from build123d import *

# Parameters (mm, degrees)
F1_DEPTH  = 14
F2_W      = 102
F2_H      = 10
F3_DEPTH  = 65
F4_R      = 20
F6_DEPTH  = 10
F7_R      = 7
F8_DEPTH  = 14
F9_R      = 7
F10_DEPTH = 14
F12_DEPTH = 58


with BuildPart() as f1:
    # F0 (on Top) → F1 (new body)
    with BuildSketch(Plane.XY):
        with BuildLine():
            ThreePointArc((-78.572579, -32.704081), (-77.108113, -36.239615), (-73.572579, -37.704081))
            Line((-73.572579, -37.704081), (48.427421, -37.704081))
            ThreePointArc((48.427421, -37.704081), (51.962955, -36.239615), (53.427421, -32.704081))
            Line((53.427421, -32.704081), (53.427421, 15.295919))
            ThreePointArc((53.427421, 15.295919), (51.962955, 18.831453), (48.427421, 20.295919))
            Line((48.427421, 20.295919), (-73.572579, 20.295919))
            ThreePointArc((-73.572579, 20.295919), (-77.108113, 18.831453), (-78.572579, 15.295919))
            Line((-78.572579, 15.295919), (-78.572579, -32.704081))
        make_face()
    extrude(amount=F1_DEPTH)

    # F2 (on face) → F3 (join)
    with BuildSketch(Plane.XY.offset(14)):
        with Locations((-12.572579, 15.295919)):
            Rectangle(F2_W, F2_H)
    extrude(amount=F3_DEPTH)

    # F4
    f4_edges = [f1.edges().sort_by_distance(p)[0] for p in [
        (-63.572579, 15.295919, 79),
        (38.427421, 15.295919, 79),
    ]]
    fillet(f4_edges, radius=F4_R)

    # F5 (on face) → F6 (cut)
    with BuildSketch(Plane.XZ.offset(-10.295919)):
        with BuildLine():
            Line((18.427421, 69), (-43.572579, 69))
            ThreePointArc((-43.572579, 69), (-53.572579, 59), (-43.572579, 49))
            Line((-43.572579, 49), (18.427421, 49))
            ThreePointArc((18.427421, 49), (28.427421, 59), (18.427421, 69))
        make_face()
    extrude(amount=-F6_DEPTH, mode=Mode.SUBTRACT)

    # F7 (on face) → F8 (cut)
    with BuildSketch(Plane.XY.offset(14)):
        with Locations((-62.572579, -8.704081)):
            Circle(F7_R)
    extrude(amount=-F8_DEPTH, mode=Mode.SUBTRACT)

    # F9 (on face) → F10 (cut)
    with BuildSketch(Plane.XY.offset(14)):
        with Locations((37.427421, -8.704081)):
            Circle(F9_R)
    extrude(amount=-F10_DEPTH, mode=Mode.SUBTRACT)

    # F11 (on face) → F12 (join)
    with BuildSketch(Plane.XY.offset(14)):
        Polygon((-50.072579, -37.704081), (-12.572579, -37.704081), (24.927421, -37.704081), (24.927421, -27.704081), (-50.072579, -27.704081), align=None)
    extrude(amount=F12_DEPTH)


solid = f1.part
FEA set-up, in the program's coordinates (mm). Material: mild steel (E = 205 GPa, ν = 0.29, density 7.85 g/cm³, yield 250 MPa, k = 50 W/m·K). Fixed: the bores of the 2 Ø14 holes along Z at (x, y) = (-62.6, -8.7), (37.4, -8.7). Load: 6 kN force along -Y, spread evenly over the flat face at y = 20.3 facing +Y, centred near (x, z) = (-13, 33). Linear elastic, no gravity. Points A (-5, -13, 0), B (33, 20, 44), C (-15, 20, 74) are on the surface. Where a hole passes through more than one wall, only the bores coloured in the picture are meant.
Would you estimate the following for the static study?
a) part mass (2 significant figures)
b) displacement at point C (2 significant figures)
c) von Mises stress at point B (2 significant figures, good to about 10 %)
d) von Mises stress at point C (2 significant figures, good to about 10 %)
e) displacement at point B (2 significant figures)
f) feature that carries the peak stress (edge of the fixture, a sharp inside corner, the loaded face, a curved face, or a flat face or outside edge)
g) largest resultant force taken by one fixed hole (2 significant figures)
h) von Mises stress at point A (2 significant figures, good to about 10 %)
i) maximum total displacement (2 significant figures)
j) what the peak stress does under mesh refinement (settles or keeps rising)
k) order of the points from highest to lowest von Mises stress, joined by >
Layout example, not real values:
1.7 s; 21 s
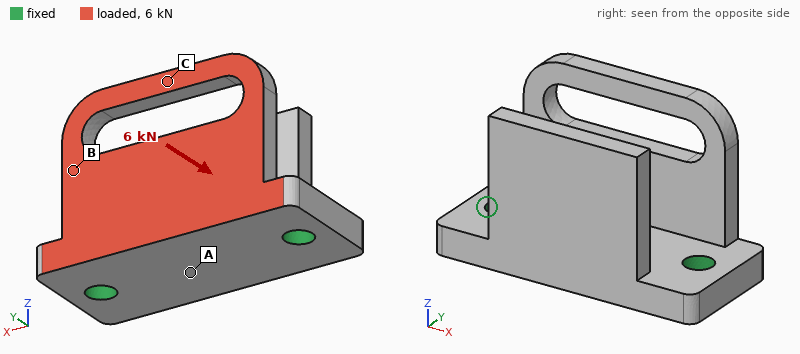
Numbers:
1.5 kg; 0.18 mm; 51 MPa; 30 MPa; 0.063 mm; a sharp inside corner; 3.0 kN; 11 MPa; 0.19 mm; keeps rising; B > C > A
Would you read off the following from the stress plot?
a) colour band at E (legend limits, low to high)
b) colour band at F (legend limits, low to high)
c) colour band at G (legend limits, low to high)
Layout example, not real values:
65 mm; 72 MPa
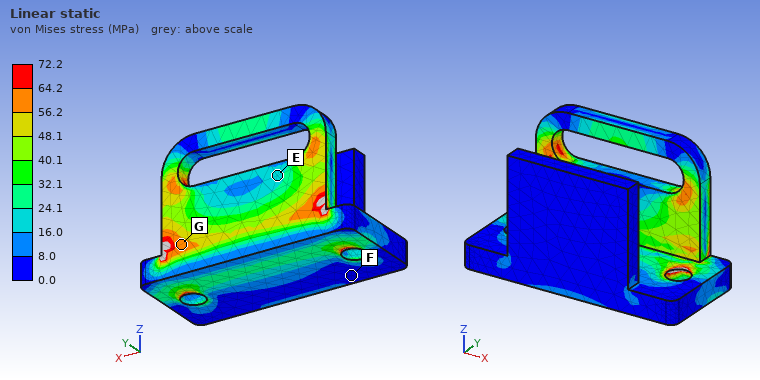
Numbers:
16.0 to 24.1 MPa; 0.0 to 8.0 MPa; 56.2 to 64.2 MPa
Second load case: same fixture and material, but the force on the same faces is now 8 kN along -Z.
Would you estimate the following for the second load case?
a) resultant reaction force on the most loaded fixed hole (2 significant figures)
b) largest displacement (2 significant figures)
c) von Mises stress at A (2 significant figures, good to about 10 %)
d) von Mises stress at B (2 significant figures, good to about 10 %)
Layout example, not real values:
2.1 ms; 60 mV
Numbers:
4.1 kN; 92 µm; 11 MPa; 25 MPa
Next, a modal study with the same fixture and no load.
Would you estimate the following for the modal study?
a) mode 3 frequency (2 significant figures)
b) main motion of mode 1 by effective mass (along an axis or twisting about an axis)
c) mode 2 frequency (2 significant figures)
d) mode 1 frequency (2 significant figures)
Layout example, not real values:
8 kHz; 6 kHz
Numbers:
3000 Hz; along Y; 1800 Hz; 1600 Hz
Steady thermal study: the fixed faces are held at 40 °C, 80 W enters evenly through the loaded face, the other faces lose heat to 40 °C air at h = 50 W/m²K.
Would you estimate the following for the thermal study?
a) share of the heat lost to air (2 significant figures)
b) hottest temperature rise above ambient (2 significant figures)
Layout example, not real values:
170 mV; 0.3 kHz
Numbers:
35 %; 58 K
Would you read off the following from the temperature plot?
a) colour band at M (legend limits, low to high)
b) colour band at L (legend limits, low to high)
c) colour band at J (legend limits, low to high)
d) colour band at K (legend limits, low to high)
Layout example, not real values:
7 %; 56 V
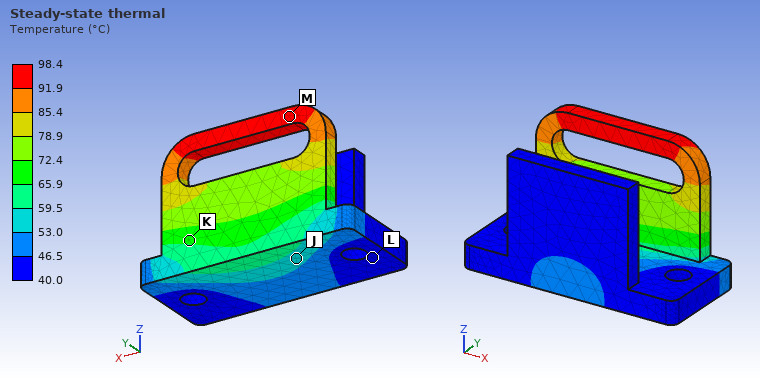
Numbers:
91.9 to 98.4 °C; 40.0 to 46.5 °C; 53.0 to 59.5 °C; 65.9 to 72.4 °C
